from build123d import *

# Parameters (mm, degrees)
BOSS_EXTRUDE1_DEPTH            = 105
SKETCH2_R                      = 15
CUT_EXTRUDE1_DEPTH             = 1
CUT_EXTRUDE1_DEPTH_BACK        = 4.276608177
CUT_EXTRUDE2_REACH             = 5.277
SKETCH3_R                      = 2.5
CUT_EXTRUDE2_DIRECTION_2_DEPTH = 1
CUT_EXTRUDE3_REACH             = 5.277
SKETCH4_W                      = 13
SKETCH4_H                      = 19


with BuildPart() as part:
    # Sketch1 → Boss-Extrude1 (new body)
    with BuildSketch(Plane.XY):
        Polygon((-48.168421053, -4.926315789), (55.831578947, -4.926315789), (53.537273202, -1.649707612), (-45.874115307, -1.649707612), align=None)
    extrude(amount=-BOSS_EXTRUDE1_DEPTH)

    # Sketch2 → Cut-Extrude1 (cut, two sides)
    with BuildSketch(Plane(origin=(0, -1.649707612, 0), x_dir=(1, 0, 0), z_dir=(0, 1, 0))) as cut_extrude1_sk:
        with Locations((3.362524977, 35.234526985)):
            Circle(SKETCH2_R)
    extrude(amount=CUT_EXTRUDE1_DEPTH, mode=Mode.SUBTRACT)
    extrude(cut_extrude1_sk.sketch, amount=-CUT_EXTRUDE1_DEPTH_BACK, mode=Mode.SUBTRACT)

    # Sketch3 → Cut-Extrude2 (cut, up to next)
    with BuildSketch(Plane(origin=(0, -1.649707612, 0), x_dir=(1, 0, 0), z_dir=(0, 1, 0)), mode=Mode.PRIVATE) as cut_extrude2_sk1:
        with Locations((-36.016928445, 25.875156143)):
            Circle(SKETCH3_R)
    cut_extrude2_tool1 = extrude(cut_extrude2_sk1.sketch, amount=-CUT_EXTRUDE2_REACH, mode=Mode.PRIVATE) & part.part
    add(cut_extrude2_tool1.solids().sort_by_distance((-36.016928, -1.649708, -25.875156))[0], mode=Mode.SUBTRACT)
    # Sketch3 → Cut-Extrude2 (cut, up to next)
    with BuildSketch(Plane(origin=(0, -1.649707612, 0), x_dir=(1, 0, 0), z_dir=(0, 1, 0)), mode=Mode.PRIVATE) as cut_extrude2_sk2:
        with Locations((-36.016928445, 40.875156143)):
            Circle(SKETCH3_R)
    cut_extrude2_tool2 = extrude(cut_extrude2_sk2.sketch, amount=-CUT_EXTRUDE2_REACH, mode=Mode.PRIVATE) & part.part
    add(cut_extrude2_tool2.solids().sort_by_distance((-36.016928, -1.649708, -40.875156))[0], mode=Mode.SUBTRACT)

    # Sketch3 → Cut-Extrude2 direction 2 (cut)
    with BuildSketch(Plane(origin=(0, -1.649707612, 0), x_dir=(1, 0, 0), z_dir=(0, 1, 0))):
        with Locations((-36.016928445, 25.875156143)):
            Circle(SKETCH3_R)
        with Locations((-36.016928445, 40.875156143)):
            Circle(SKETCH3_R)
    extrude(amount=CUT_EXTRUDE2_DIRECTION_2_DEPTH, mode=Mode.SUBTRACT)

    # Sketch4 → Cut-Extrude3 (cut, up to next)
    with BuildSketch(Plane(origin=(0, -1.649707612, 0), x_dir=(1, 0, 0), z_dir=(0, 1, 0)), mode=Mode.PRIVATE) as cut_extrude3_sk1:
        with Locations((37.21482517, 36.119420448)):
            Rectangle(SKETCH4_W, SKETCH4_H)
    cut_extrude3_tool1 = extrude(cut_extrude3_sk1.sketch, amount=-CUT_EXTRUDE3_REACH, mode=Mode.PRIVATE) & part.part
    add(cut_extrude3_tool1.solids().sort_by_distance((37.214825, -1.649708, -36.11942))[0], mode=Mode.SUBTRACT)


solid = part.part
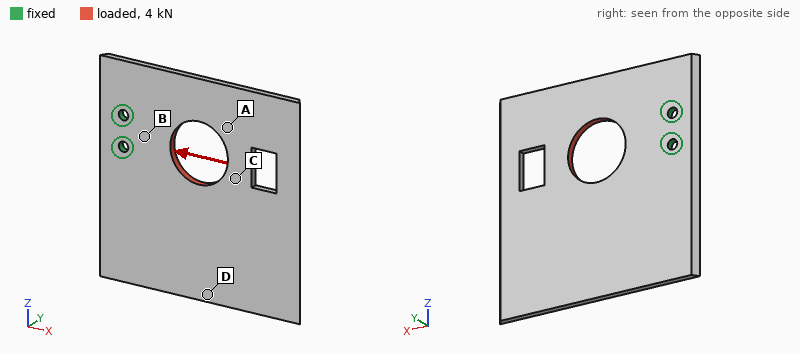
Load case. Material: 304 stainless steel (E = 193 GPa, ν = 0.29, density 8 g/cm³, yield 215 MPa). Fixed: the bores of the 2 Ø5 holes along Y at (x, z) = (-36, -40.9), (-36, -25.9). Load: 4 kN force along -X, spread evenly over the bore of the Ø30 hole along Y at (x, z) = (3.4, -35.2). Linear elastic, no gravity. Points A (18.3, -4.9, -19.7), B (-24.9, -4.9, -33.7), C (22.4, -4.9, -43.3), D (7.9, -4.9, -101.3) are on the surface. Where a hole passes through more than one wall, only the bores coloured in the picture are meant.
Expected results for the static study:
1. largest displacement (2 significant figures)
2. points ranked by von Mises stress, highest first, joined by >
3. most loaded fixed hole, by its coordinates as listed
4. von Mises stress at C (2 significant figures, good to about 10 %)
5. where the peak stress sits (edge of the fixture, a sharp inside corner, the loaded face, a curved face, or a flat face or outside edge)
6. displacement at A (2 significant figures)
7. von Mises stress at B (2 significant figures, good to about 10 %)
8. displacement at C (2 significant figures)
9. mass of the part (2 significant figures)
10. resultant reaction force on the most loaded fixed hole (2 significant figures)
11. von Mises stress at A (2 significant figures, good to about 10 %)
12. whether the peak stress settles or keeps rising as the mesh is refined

13 µm
B > C > A > D
(-36, -40.9)
19 MPa
edge of the fixture
9.0 µm
25 MPa
12 µm
250 g
2.4 kN
9.4 MPa
keeps rising
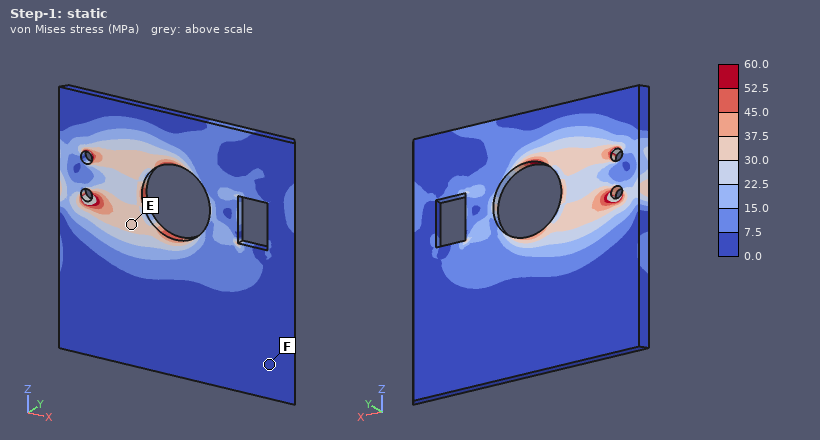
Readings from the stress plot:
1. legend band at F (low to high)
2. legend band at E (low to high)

0.0 to 7.5 MPa
30.0 to 37.5 MPa
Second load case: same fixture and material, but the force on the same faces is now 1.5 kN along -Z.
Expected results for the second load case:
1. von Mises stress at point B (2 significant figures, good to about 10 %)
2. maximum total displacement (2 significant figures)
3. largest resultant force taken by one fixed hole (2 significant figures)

59 MPa
69 µm
3.0 kN
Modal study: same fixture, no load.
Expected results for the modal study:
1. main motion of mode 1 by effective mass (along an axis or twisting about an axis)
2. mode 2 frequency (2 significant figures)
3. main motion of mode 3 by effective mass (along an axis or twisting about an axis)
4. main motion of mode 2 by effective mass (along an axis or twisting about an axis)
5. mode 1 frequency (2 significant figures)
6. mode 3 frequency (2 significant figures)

along Y
430 Hz
along Y
twisting about X
240 Hz
920 Hz
